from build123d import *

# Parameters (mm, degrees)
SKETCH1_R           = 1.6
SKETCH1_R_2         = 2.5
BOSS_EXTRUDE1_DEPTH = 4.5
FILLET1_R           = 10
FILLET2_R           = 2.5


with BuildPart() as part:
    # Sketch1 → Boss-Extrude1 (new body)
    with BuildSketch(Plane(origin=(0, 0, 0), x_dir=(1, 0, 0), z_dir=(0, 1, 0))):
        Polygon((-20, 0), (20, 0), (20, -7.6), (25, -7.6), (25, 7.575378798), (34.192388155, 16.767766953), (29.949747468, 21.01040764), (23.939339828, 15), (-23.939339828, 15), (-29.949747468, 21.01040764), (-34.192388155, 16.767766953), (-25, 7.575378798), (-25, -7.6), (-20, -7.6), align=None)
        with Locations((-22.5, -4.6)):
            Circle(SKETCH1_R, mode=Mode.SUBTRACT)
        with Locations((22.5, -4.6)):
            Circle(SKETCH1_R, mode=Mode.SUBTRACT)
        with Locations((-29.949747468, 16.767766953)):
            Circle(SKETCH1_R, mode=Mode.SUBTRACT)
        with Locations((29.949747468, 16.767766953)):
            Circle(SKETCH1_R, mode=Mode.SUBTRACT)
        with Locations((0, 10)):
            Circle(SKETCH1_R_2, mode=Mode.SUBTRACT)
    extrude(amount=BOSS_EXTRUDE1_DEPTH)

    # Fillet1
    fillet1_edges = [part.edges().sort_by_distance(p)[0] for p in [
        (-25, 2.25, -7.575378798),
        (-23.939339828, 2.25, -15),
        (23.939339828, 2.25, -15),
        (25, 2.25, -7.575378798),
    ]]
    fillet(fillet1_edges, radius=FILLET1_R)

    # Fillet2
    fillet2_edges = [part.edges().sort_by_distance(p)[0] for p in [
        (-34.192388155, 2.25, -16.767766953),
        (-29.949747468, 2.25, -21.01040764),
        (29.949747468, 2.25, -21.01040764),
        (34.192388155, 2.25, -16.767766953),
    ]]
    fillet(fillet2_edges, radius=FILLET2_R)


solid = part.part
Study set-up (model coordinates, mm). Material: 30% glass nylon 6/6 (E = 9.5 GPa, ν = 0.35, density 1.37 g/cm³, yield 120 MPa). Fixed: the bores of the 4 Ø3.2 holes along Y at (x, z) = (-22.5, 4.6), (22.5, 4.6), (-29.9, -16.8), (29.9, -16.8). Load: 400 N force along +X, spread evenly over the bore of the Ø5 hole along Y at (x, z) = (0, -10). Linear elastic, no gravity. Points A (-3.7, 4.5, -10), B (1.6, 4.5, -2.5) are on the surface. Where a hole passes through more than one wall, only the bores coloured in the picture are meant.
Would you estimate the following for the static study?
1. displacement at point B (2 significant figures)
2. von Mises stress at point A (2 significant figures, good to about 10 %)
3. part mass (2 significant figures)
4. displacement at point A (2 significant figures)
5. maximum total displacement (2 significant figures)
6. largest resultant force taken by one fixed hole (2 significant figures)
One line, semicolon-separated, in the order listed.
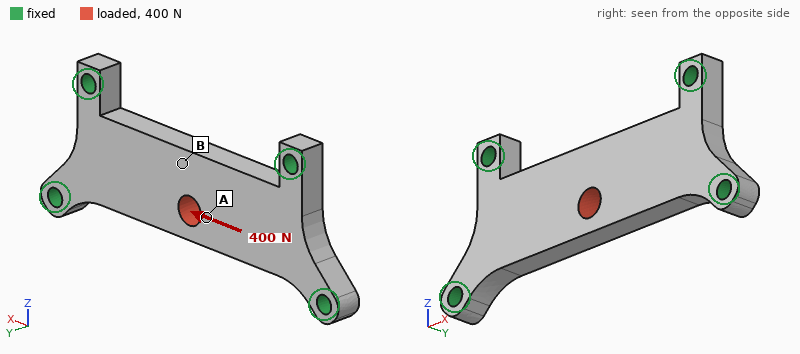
10 µm; 5.9 MPa; 5.5 g; 14 µm; 16 µm; 140 N
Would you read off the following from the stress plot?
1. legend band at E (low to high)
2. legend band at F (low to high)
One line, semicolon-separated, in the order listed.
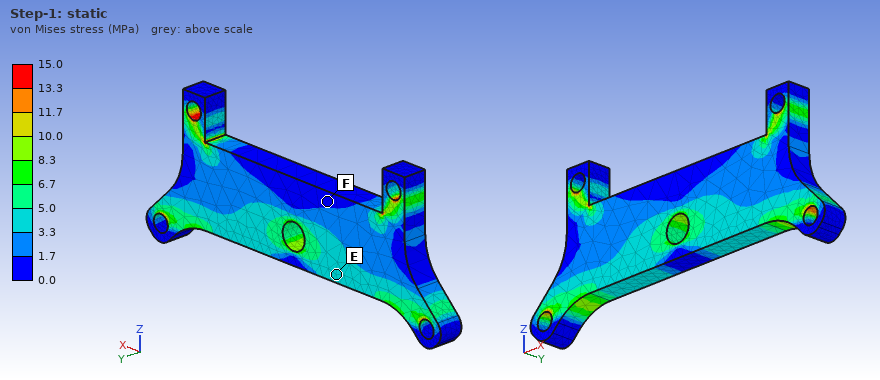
3.3 to 5.0 MPa; 0.0 to 1.7 MPa
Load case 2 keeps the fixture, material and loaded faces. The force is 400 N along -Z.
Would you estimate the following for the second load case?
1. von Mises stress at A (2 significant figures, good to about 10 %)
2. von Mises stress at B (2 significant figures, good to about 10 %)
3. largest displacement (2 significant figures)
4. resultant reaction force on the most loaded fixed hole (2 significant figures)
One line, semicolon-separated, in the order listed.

7.9 MPa; 9.0 MPa; 50 µm; 180 N
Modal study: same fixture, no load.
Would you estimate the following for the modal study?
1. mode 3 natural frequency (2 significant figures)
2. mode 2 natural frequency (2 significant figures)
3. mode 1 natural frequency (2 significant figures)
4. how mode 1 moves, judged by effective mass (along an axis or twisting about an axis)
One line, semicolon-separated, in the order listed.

9100 Hz; 9100 Hz; 3400 Hz; along Y
